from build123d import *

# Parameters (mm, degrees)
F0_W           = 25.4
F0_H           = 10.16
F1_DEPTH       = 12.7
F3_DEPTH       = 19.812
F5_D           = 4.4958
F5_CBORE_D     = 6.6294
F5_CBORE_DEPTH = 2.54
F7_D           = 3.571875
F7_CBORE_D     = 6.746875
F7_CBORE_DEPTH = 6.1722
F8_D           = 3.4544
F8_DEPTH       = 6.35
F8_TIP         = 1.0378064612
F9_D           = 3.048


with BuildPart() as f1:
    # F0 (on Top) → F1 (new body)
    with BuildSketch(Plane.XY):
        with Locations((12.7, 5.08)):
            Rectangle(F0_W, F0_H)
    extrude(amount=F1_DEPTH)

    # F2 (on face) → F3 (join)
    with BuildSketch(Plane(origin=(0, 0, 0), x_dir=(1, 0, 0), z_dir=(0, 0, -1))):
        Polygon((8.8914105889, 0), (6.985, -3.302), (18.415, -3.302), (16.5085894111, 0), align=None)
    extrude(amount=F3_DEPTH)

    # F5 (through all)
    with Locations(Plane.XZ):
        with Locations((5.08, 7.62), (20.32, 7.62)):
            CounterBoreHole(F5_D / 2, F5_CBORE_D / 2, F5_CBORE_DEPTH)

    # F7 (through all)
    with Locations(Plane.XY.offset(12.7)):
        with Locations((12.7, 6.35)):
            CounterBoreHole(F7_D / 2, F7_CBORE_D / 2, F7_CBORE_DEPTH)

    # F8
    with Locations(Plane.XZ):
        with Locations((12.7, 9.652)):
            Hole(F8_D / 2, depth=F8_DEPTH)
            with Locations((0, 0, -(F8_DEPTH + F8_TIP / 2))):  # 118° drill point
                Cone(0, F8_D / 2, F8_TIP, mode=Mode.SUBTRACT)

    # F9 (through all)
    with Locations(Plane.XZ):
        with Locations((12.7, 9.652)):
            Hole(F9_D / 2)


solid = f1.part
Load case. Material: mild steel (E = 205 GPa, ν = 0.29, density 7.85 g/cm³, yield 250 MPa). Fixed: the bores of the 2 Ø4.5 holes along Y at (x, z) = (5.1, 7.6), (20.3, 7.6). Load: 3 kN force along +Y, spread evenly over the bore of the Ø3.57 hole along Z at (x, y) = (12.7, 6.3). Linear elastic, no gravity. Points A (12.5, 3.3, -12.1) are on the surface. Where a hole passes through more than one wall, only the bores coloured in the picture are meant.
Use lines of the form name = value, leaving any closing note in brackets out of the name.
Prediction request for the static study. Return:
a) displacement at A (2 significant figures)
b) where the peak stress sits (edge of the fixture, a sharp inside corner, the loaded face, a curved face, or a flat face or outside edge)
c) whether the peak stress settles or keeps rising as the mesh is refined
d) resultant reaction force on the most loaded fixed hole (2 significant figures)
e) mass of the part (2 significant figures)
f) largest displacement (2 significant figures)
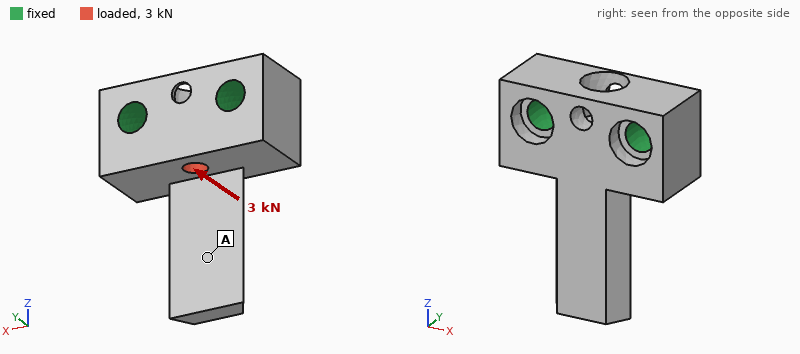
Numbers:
displacement at A = 6.3 µm
where the peak stress sits = edge of the fixture
whether the peak stress settles or keeps rising as the mesh is refined = keeps rising
resultant reaction force on the most loaded fixed hole = 1.5 kN
mass of the part = 25 g
largest displacement = 8.7 µm
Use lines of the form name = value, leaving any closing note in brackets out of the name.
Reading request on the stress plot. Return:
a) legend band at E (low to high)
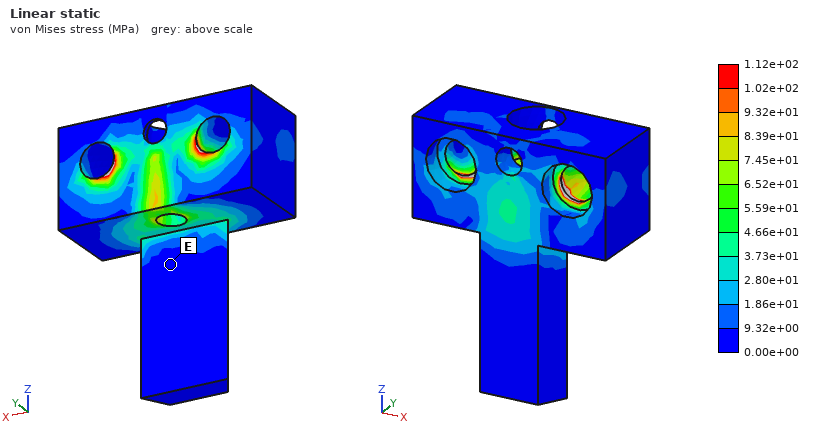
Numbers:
legend band at E = 0.00e+00 to 9.32e+00 MPa
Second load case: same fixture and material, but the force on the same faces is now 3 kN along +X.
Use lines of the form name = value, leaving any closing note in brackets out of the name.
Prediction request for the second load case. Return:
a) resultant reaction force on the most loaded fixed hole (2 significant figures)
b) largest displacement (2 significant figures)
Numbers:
resultant reaction force on the most loaded fixed hole = 1.6 kN
largest displacement = 1.6 µm
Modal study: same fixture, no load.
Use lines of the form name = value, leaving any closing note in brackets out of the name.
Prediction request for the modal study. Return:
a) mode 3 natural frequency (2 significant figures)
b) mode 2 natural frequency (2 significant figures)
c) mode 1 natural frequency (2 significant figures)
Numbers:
mode 3 natural frequency = 23 kHz
mode 2 natural frequency = 14 kHz
mode 1 natural frequency = 5700 Hz
